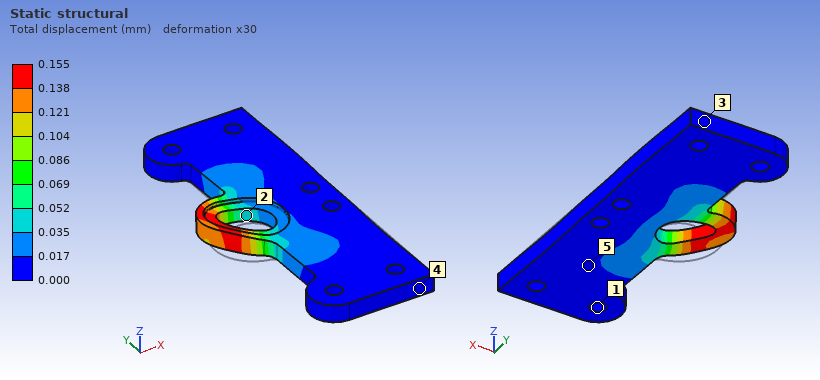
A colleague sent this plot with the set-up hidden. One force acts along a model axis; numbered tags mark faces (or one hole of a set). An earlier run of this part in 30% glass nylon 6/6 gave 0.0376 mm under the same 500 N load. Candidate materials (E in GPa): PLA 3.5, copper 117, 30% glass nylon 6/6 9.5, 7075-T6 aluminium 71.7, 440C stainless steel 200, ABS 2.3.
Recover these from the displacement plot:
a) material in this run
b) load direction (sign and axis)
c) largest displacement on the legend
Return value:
ABS
+Y
0.155 mm
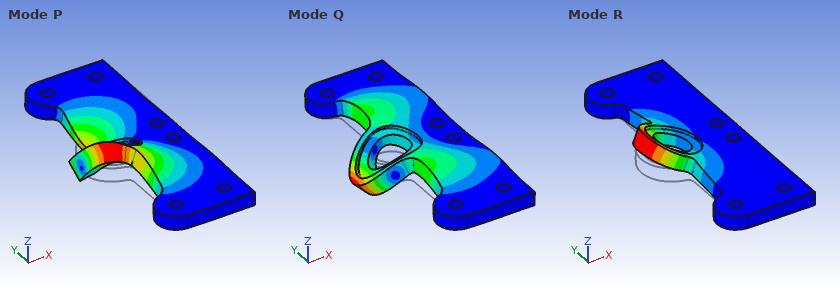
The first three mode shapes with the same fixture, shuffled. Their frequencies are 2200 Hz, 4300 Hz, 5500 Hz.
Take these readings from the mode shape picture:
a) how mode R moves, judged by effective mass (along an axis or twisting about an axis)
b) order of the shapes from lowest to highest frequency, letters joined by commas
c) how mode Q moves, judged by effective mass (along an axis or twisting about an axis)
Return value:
along Z
R, P, Q
along Z
